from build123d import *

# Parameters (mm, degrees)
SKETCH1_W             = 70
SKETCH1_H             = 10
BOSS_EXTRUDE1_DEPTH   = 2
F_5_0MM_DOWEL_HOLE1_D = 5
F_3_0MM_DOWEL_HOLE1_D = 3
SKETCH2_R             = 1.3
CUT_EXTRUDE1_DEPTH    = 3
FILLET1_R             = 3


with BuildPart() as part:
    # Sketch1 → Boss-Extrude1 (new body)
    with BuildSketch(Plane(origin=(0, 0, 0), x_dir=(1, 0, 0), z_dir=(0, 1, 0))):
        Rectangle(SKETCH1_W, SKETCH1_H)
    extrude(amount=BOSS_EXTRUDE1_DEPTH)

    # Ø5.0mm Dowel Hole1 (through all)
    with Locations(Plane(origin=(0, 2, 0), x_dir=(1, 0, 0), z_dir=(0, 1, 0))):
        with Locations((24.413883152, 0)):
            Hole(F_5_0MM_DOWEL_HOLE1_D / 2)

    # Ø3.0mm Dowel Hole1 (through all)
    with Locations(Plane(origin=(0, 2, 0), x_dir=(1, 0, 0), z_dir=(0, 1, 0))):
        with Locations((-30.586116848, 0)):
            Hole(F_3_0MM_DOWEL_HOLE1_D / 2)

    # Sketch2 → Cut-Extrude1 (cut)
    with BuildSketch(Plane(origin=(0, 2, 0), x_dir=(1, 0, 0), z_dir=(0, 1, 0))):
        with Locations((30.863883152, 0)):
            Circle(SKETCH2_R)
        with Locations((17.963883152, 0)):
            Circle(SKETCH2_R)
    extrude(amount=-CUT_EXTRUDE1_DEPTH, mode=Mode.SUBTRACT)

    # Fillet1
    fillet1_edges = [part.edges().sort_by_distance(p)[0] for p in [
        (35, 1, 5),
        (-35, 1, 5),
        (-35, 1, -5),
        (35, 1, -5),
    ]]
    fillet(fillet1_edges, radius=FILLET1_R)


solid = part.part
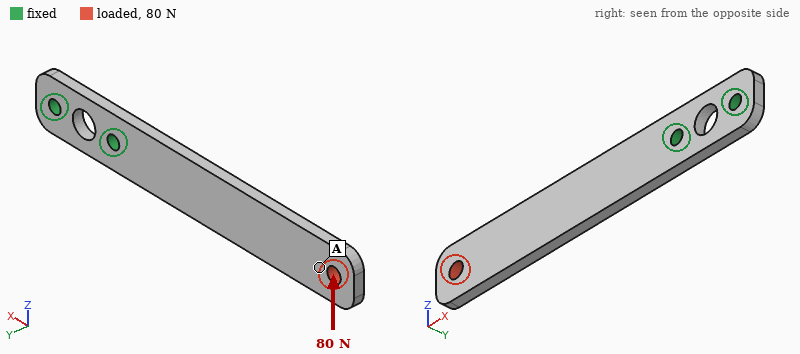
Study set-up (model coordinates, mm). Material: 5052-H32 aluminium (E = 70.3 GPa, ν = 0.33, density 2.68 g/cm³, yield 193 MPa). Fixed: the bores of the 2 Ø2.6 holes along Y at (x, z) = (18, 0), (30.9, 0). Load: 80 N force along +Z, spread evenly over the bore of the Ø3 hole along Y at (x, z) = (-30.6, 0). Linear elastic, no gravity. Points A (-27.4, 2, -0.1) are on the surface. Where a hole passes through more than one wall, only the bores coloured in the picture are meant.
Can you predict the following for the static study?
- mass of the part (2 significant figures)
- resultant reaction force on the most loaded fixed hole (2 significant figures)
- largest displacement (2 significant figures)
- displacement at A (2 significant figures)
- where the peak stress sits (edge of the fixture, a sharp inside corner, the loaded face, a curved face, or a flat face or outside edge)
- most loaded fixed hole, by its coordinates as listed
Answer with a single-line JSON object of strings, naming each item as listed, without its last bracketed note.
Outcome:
{"mass of the part": "3.5 g", "resultant reaction force on the most loaded fixed hole": "210 N", "largest displacement": "0.38 mm", "displacement at A": "0.31 mm", "where the peak stress sits": "edge of the fixture", "most loaded fixed hole, by its coordinates as listed": "(18, 0)"}
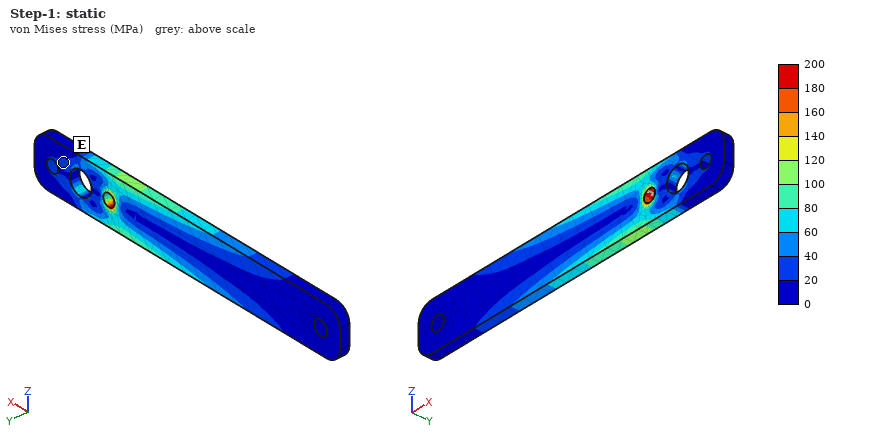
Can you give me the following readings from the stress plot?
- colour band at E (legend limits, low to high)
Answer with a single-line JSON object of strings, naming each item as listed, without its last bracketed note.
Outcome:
{"colour band at E": "20 to 40 MPa"}
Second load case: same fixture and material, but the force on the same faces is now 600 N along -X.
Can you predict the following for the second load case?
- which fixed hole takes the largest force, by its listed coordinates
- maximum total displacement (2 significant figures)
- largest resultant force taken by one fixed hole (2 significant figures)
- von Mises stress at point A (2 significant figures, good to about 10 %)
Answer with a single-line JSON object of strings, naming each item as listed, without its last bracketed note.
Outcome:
{"which fixed hole takes the largest force, by its listed coordinates": "(18, 0)", "maximum total displacement": "24 µm", "largest resultant force taken by one fixed hole": "540 N", "von Mises stress at point A": "35 MPa"}
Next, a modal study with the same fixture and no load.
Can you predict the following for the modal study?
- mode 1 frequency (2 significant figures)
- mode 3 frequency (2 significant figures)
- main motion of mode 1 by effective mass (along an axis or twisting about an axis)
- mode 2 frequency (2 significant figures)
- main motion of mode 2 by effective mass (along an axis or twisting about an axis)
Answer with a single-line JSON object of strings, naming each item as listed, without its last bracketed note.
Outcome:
{"mode 1 frequency": "630 Hz", "mode 3 frequency": "3800 Hz", "main motion of mode 1 by effective mass": "along Y", "mode 2 frequency": "2600 Hz", "main motion of mode 2 by effective mass": "along Z"}
